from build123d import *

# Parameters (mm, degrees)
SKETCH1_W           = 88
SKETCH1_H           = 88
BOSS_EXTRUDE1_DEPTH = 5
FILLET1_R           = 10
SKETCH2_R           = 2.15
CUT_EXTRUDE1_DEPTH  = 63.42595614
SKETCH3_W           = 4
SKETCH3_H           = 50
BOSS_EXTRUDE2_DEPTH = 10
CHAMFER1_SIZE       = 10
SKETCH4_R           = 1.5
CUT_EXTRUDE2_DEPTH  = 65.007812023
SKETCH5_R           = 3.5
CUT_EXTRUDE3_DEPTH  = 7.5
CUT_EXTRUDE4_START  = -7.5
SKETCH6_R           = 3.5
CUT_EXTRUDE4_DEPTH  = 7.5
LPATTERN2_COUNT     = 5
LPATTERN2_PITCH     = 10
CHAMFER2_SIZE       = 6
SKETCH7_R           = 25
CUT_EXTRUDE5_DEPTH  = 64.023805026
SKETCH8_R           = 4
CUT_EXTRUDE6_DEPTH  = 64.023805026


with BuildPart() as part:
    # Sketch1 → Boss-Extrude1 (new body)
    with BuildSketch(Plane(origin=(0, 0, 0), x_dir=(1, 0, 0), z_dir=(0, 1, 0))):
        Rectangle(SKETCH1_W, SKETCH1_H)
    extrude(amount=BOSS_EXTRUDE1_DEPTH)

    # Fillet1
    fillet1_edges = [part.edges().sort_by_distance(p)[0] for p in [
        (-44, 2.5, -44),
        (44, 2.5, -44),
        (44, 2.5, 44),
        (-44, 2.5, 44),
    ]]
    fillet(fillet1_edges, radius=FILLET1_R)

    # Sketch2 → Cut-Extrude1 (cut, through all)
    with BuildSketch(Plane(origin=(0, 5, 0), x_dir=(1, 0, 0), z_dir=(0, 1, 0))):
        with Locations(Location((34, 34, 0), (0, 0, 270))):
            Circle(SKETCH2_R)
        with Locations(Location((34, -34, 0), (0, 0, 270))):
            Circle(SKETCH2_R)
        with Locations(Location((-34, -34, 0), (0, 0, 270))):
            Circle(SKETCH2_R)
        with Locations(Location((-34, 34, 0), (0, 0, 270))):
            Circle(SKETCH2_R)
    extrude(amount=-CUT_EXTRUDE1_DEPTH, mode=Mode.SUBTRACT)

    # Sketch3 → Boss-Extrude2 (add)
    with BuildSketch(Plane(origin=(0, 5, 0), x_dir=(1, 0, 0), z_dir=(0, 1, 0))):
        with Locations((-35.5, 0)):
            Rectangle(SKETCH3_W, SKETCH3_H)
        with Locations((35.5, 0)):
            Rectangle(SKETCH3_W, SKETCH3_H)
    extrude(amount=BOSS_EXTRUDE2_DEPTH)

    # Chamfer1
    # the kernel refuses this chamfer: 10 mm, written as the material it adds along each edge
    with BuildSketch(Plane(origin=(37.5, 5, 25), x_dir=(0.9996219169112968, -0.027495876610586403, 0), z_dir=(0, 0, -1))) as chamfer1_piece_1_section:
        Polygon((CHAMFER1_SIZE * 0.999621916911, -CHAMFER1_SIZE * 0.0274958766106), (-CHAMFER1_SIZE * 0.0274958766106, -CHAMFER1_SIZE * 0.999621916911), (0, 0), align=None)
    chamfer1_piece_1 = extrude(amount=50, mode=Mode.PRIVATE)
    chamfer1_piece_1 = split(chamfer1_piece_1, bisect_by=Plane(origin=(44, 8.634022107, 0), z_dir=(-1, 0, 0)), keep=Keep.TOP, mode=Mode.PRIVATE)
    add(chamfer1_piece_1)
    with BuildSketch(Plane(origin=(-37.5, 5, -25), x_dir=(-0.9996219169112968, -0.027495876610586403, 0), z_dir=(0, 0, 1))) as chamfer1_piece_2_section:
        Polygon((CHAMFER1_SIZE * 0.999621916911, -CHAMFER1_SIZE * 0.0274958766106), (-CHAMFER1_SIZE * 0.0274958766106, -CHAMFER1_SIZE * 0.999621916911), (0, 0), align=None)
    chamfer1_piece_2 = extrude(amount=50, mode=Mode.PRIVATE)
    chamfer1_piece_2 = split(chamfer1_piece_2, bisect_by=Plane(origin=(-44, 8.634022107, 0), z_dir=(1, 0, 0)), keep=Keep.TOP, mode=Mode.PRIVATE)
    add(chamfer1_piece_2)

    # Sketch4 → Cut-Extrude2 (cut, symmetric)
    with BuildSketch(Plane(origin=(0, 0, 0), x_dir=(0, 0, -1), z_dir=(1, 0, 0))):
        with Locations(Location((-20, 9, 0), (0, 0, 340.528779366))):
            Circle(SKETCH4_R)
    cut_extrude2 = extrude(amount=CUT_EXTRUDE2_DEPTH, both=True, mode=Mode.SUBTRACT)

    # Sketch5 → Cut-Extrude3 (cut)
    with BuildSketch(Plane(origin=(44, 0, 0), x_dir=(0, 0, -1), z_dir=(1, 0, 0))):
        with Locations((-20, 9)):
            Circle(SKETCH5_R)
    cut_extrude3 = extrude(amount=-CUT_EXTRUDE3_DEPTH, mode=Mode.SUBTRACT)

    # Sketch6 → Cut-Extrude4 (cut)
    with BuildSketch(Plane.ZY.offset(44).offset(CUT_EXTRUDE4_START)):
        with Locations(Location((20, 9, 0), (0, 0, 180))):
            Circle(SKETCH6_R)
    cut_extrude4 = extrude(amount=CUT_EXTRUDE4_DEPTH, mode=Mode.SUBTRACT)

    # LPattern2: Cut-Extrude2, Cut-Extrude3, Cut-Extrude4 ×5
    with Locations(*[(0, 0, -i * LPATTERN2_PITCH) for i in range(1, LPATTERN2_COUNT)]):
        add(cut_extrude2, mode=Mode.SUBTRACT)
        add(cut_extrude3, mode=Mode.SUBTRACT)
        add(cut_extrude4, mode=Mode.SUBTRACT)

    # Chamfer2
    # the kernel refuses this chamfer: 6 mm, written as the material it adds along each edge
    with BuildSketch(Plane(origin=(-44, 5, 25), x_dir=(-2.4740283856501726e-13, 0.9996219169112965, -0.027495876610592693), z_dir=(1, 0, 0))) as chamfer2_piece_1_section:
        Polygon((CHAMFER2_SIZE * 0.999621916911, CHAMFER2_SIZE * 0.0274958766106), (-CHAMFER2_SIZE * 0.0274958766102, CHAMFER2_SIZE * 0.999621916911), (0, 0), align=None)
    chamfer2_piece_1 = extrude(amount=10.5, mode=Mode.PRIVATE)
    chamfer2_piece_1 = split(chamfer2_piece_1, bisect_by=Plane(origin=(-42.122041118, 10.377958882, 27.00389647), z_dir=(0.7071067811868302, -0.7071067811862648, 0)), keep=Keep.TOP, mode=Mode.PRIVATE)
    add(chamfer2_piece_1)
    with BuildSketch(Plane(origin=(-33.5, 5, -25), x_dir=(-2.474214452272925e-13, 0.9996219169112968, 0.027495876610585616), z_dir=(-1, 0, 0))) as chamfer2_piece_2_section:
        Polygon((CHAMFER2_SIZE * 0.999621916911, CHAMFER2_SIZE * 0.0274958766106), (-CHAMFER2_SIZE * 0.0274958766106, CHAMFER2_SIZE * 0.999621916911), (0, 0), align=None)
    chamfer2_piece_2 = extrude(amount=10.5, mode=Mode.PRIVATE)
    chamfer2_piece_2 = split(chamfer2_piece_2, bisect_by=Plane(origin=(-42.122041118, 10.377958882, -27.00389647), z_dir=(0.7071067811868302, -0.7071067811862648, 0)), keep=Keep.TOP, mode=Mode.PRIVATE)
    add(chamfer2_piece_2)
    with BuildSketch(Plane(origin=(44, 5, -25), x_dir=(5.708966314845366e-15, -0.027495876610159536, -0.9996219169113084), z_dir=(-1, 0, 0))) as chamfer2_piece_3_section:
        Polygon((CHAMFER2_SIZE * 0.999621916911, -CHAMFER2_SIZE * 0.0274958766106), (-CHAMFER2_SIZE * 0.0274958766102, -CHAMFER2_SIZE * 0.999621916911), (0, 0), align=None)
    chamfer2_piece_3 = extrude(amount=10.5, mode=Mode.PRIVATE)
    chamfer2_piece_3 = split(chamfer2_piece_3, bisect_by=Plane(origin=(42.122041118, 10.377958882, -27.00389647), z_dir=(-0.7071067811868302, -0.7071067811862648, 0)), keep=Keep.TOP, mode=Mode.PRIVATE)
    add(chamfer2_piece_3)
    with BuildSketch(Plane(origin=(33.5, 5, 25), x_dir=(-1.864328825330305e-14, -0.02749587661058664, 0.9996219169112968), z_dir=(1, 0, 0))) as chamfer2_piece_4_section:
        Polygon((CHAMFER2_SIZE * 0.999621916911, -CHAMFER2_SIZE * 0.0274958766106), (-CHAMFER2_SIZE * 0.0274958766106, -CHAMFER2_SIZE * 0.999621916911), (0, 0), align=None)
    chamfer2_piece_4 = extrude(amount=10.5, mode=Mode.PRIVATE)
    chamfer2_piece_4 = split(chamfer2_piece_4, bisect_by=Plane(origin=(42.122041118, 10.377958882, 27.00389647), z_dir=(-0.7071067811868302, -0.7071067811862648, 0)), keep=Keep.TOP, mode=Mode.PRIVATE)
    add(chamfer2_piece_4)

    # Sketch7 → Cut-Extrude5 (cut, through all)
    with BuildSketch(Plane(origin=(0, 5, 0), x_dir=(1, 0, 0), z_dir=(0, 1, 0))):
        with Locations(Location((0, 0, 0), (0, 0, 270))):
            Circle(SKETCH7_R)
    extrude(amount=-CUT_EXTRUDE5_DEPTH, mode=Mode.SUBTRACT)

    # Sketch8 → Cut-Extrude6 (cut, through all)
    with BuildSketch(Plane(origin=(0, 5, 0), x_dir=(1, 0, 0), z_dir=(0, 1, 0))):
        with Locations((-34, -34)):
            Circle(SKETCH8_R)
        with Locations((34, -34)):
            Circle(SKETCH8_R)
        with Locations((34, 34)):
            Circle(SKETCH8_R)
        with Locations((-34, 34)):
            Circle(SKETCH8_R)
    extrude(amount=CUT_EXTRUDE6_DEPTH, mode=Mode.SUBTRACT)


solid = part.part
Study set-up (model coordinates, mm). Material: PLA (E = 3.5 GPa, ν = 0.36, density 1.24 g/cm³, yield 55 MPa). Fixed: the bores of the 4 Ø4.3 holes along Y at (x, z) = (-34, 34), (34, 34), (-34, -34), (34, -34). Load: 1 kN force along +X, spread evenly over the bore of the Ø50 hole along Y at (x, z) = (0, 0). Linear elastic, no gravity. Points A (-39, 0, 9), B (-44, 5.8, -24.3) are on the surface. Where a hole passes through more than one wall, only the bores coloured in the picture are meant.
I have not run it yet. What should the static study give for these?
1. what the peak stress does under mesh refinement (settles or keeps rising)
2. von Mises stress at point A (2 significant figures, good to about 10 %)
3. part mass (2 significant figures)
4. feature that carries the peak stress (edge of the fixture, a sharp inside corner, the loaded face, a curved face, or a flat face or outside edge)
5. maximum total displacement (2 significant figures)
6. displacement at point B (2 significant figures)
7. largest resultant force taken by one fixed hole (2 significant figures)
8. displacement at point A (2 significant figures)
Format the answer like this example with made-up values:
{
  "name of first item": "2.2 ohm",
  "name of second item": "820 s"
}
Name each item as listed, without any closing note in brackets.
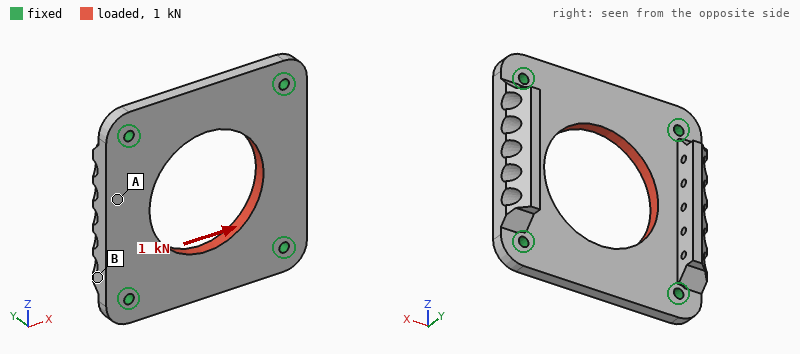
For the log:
{
  "what the peak stress does under mesh refinement": "keeps rising",
  "von Mises stress at point A": "1.6 MPa",
  "part mass": "43 g",
  "feature that carries the peak stress": "edge of the fixture",
  "maximum total displacement": "48 µm",
  "displacement at point B": "20 µm",
  "largest resultant force taken by one fixed hole": "260 N",
  "displacement at point A": "39 µm"
}
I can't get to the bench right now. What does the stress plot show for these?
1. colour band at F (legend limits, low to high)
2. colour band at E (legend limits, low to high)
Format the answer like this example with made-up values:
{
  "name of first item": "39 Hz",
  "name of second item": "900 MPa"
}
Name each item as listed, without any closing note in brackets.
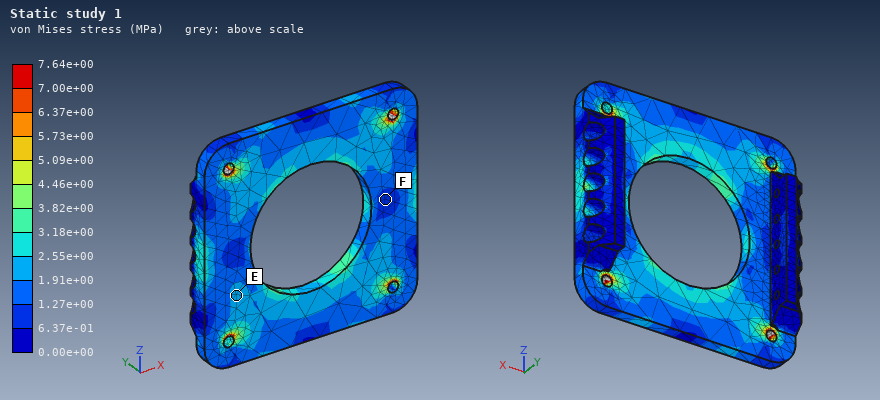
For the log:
{
  "colour band at F": "6.37e-01 to 1.27e+00 MPa",
  "colour band at E": "1.91e+00 to 2.55e+00 MPa"
}
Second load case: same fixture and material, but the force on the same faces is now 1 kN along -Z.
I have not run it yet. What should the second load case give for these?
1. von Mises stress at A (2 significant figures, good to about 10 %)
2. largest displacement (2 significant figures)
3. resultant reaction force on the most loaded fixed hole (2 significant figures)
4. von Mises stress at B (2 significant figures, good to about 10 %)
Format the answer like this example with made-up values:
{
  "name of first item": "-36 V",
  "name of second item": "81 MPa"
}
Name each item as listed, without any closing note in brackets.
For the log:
{
  "von Mises stress at A": "1.3 MPa",
  "largest displacement": "47 µm",
  "resultant reaction force on the most loaded fixed hole": "260 N",
  "von Mises stress at B": "0.81 MPa"
}
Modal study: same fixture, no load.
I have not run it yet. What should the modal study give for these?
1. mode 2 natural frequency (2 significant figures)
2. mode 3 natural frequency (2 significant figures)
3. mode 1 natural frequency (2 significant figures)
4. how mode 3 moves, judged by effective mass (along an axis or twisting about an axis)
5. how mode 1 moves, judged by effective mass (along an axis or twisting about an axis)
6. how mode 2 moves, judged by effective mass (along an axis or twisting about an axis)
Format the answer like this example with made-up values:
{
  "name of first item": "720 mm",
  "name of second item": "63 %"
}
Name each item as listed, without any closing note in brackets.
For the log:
{
  "mode 2 natural frequency": "1900 Hz",
  "mode 3 natural frequency": "2400 Hz",
  "mode 1 natural frequency": "1800 Hz",
  "how mode 3 moves, judged by effective mass": "along Y",
  "how mode 1 moves, judged by effective mass": "along Y",
  "how mode 2 moves, judged by effective mass": "twisting about X"
}
